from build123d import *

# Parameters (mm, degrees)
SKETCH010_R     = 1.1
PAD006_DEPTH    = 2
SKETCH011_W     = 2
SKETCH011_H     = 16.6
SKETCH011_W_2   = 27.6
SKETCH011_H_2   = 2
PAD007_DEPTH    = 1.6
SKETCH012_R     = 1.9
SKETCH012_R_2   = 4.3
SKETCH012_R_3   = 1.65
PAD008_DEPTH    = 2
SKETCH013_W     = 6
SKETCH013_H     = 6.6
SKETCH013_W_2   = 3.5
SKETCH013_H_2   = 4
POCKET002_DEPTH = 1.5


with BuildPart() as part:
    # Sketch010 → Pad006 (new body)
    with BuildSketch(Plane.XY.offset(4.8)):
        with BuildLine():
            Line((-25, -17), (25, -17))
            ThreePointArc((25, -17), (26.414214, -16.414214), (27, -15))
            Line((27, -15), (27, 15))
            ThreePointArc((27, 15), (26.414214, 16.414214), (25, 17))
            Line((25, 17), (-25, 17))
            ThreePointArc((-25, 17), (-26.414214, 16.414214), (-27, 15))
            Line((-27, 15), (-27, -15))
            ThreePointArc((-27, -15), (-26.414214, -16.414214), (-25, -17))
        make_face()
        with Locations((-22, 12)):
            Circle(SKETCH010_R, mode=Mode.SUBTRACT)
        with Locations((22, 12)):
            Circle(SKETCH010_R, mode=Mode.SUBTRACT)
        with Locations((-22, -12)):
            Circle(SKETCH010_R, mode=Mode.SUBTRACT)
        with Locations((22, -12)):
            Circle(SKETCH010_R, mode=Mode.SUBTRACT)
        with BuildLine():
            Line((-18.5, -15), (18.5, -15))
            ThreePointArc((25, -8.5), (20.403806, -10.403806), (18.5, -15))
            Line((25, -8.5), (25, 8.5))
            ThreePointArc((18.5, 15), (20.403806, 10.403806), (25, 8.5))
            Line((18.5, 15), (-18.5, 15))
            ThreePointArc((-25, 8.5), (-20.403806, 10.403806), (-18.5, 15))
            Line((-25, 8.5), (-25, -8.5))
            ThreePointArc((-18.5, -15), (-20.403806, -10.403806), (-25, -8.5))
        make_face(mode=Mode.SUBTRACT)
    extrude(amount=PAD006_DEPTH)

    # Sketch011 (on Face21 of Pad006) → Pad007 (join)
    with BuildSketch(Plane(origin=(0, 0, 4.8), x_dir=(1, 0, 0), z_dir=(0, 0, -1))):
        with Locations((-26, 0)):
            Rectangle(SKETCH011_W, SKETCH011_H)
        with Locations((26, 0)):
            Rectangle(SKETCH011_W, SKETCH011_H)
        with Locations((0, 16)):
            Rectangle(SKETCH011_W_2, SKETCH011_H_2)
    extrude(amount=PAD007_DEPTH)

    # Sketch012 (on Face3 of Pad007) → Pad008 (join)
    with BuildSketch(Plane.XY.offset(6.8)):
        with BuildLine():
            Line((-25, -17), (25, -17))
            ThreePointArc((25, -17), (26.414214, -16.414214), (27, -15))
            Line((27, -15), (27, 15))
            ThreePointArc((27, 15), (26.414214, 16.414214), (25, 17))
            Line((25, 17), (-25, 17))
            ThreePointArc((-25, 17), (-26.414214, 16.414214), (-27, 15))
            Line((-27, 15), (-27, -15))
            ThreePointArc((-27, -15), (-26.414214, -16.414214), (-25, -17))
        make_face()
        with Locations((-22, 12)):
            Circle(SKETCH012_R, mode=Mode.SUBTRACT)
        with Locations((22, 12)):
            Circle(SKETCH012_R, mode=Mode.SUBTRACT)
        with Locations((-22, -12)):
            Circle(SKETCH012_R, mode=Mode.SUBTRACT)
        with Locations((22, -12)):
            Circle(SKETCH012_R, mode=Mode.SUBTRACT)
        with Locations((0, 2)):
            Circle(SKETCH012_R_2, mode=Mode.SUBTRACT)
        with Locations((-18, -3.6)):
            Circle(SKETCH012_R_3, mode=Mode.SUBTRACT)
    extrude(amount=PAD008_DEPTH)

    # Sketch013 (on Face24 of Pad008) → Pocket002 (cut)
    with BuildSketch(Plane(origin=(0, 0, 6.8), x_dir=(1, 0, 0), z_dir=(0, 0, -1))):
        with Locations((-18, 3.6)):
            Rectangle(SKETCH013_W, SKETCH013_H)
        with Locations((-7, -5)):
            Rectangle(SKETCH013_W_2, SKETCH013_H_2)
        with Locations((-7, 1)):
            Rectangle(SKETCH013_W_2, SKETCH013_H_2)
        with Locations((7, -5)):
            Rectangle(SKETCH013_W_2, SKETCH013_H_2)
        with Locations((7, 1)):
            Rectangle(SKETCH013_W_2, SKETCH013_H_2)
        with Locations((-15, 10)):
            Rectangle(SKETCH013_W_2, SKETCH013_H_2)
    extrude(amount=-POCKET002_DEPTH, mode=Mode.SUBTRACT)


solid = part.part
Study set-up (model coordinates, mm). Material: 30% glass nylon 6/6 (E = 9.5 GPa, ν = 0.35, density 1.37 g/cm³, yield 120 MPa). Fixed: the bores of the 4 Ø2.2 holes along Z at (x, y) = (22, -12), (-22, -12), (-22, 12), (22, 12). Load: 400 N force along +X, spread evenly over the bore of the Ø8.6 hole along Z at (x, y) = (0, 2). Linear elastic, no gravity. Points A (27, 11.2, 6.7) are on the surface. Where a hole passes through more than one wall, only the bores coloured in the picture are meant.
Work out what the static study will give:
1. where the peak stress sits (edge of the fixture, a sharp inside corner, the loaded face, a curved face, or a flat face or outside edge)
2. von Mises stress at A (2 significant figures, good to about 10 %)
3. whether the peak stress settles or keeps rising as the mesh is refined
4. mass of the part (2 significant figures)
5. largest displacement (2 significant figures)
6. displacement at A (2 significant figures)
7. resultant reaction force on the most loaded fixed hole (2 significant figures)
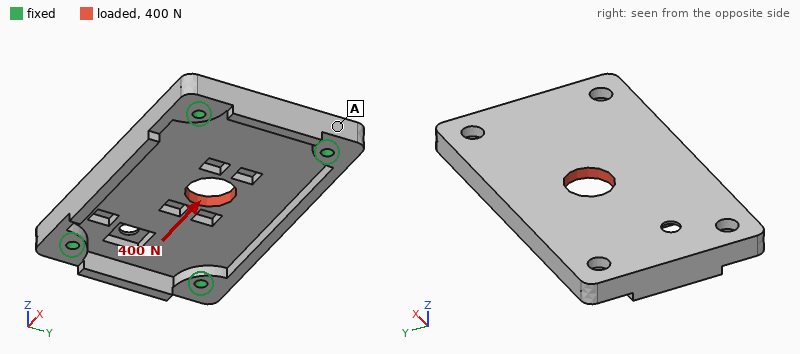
edge of the fixture
3.2 MPa
keeps rising
6.0 g
26 µm
9.4 µm
110 N
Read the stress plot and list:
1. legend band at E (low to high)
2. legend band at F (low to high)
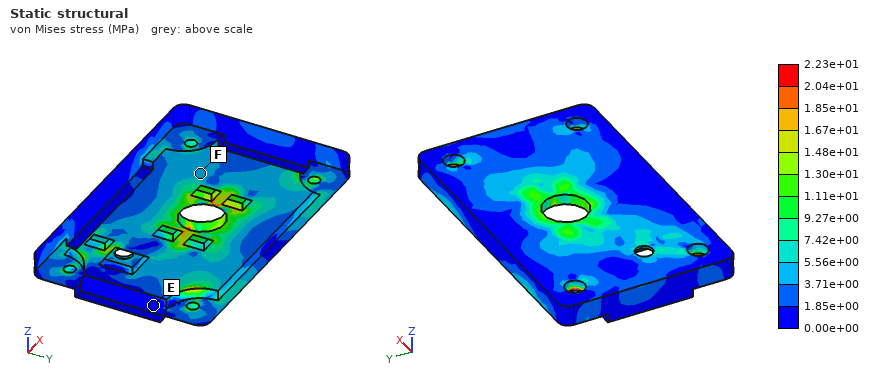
0.00e+00 to 1.85e+00 MPa
3.71e+00 to 5.56e+00 MPa
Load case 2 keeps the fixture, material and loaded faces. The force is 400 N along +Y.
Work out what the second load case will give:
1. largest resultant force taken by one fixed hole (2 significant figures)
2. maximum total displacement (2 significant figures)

120 N
47 µm
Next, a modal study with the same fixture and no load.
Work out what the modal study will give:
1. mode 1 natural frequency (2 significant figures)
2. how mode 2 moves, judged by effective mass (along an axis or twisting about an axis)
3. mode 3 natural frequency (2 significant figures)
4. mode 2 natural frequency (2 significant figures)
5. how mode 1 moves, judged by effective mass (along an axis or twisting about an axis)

3300 Hz
twisting about X
6400 Hz
4600 Hz
along Z
